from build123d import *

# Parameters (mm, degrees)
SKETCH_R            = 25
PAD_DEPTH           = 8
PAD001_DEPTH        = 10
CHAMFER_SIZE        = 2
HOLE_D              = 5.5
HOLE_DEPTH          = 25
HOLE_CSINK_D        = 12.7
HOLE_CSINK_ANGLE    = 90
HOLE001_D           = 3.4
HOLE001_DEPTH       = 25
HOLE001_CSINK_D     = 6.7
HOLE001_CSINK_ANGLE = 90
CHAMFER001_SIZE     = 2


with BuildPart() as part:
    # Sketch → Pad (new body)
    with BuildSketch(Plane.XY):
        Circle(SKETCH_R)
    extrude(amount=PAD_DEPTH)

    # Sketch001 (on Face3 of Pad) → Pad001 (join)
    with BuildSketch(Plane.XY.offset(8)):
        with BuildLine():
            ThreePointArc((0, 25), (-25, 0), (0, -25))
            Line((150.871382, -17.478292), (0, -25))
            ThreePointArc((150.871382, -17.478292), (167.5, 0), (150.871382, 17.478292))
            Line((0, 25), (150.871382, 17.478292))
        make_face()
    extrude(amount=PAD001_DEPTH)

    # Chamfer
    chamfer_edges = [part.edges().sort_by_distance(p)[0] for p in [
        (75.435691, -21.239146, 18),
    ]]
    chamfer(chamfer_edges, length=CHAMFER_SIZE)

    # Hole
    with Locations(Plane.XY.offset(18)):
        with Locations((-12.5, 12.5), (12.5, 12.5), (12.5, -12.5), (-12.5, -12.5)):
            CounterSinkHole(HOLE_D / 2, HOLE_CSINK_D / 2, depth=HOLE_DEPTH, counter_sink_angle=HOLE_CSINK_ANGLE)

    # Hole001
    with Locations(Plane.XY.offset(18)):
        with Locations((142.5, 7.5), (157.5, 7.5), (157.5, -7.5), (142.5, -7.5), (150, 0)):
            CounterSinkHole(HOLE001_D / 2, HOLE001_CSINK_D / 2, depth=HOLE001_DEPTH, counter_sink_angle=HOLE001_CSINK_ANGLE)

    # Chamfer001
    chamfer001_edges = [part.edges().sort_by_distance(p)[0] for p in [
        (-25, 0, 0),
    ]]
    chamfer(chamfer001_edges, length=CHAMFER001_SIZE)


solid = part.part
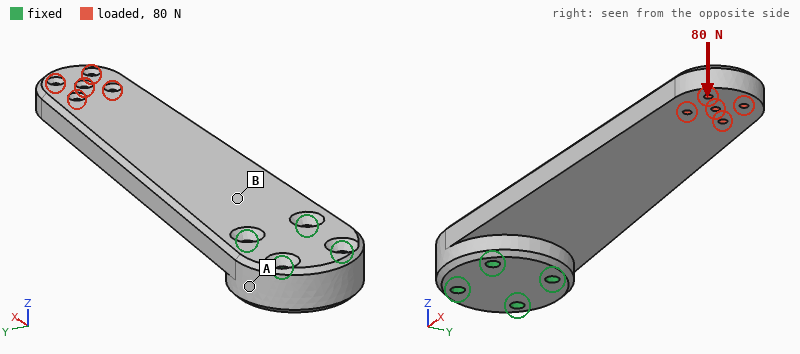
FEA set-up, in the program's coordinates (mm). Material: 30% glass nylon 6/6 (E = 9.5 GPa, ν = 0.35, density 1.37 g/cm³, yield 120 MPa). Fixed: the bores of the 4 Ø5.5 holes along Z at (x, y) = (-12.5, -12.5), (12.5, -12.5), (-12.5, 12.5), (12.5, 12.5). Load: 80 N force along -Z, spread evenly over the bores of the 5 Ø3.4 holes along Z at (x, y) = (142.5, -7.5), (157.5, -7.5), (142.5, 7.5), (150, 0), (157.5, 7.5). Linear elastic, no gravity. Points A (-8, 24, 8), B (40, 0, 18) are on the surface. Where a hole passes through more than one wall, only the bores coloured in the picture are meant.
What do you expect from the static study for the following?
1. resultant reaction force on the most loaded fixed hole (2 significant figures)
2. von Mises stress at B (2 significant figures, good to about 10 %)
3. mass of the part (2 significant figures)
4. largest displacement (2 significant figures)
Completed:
130 N
11 MPa
120 g
2.2 mm
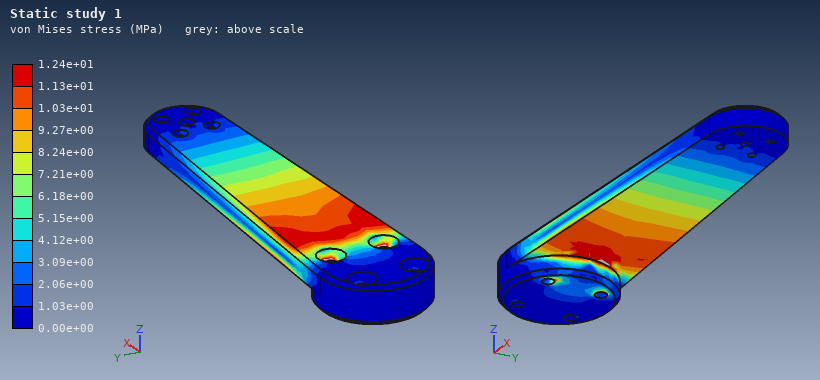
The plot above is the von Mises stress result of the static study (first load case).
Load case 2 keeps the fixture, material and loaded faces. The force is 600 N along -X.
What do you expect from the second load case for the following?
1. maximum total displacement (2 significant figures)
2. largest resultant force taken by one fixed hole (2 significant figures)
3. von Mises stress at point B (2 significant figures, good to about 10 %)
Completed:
0.13 mm
250 N
0.82 MPa
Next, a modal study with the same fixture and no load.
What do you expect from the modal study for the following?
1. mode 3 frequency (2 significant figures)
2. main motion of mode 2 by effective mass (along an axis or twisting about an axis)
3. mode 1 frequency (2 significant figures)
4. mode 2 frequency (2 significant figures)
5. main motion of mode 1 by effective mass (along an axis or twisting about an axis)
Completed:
1200 Hz
along Y
220 Hz
860 Hz
along Z
